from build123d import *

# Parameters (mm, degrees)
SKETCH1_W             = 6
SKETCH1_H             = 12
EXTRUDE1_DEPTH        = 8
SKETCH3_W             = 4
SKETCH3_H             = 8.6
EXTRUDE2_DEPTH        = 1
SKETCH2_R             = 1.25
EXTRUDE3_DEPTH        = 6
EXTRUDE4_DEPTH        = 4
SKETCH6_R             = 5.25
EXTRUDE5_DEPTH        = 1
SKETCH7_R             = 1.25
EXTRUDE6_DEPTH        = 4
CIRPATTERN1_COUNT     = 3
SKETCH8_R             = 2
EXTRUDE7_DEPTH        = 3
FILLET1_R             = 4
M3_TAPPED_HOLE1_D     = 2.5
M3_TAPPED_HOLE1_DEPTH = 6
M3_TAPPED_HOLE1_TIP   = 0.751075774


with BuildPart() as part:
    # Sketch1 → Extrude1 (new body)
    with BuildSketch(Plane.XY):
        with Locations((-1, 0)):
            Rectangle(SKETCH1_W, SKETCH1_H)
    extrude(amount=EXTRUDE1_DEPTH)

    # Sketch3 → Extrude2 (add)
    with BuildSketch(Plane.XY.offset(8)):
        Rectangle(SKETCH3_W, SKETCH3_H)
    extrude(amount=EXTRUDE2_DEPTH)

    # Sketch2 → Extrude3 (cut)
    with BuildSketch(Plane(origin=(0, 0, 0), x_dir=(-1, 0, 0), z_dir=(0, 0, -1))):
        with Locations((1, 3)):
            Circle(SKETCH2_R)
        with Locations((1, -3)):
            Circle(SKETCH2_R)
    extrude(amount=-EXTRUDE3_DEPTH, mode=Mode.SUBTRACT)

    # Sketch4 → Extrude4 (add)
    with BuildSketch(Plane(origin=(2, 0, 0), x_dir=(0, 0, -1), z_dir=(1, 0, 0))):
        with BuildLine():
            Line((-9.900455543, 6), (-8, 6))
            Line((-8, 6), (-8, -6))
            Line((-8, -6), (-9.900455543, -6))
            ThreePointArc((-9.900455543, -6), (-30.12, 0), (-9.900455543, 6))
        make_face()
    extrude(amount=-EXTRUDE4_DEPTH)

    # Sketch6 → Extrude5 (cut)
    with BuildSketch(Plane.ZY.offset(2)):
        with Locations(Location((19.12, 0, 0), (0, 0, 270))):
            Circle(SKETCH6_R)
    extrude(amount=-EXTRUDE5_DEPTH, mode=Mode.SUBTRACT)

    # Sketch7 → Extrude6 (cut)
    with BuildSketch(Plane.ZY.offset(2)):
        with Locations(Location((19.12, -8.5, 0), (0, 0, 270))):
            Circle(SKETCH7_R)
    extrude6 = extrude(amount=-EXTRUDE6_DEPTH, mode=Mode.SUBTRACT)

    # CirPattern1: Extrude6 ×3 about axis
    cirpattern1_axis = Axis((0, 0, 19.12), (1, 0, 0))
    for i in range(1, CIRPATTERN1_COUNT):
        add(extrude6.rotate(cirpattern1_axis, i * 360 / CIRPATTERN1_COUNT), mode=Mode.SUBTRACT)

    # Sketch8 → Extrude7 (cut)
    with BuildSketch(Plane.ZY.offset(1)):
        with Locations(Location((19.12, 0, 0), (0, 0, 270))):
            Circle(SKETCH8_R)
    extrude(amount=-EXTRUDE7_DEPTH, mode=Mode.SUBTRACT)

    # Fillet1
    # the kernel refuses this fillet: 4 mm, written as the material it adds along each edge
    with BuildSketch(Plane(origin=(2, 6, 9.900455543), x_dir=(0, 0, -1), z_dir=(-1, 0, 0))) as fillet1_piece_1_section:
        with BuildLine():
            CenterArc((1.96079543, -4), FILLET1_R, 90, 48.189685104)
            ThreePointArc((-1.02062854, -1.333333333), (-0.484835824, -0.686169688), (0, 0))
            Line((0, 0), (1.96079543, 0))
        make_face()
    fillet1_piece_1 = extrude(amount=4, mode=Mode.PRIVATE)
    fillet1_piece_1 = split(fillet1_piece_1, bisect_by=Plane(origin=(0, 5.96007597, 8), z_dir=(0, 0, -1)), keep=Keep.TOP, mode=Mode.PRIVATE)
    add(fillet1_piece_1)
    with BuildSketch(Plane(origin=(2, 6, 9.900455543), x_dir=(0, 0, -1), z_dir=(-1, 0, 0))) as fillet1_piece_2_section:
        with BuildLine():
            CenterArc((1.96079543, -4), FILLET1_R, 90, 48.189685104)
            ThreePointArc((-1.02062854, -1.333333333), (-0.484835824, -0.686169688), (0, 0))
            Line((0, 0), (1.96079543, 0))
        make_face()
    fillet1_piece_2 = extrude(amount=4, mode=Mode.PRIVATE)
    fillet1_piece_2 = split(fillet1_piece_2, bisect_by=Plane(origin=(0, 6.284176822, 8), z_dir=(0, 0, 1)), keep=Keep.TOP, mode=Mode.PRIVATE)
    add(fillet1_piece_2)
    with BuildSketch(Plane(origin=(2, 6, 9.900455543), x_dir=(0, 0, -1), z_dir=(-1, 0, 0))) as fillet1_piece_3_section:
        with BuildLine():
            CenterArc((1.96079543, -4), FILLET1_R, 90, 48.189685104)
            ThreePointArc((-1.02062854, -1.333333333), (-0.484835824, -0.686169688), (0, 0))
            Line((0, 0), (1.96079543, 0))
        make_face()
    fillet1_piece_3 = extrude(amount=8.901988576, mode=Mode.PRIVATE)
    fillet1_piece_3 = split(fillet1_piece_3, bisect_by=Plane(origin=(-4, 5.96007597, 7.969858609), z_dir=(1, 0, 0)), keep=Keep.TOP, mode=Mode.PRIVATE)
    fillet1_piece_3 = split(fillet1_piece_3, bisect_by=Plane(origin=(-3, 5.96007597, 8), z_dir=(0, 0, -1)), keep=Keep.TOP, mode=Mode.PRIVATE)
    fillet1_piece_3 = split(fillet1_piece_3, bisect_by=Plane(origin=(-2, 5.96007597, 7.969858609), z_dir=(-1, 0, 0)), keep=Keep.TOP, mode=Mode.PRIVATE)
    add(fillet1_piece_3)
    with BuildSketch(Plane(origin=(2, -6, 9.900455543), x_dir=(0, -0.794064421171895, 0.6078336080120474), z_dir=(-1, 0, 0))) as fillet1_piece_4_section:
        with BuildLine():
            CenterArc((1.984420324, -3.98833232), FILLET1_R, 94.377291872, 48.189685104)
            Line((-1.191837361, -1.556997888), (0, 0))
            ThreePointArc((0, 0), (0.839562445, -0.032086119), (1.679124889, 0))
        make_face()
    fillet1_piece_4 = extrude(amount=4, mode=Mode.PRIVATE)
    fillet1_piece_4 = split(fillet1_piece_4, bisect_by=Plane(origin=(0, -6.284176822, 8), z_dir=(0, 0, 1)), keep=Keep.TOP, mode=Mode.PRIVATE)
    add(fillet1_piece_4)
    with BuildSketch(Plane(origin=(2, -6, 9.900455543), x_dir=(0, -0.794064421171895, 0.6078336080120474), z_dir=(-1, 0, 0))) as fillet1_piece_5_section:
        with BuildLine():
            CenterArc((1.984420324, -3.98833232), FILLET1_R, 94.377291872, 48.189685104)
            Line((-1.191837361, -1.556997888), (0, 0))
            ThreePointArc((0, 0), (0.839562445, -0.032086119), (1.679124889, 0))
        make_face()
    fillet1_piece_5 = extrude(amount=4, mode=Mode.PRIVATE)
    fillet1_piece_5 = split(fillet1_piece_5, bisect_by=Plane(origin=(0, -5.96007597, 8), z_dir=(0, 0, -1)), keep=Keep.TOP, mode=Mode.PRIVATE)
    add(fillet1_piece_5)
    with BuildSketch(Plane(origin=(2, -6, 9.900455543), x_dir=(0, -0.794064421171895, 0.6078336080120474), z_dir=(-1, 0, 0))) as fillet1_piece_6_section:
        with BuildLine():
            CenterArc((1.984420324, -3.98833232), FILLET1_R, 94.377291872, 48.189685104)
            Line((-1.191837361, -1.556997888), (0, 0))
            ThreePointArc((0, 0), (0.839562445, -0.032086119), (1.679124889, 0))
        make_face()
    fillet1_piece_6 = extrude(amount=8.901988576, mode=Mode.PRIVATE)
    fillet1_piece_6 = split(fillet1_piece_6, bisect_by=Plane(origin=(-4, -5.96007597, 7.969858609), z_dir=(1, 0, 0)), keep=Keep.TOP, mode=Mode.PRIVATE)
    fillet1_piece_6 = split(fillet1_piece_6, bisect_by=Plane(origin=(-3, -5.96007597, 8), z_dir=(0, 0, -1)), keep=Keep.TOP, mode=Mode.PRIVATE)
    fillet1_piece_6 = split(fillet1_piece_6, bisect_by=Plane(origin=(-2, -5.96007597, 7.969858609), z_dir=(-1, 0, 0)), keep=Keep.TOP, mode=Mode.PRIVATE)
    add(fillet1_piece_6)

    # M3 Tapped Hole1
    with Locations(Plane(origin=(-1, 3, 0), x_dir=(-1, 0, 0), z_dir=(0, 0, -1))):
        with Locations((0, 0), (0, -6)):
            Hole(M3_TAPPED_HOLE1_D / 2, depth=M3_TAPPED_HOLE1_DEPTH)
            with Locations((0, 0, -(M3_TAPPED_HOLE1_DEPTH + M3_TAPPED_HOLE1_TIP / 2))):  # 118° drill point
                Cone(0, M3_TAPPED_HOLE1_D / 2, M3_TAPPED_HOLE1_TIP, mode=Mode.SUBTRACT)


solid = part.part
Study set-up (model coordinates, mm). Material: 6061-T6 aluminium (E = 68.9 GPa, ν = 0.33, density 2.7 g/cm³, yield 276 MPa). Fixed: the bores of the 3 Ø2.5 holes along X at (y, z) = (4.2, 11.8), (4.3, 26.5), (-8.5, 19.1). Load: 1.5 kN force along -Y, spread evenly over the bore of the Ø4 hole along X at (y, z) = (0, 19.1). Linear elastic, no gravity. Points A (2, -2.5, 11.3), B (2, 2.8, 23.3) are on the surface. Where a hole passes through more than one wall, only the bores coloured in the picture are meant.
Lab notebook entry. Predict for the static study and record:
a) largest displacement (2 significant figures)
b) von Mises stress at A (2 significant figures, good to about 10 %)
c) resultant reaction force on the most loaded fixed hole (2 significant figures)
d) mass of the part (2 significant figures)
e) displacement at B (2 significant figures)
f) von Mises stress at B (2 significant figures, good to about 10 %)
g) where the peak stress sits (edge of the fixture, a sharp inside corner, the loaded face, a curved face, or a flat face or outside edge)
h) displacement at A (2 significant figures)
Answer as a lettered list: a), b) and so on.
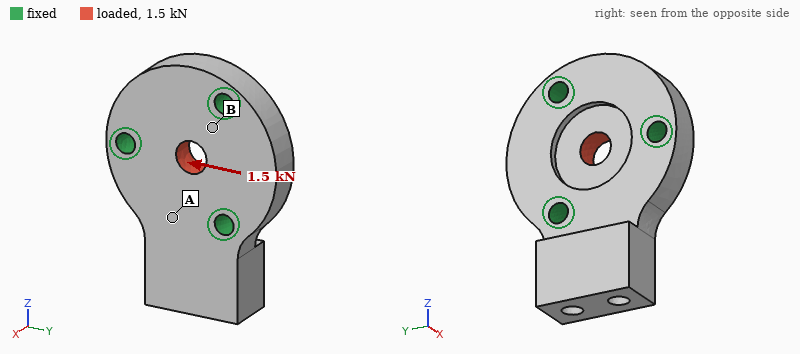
a) 4.4 µm
b) 7.9 MPa
c) 530 N
d) 5.1 g
e) 1.6 µm
f) 22 MPa
g) the loaded face
h) 1.0 µm
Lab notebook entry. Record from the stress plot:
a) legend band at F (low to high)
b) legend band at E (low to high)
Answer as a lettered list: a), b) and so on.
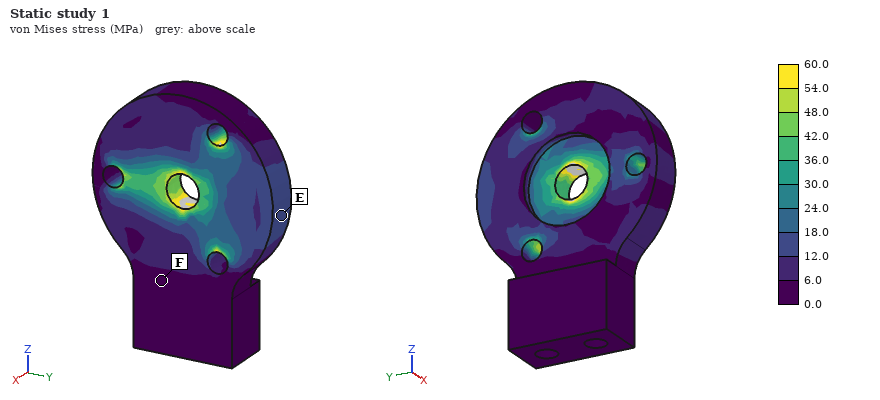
a) 0.0 to 6.0 MPa
b) 12.0 to 18.0 MPa
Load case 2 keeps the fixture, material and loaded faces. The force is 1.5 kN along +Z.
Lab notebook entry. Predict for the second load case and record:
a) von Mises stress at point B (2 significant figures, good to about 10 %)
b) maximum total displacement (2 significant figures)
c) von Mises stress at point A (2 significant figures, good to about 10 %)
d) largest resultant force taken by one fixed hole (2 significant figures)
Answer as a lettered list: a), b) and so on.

a) 34 MPa
b) 4.1 µm
c) 13 MPa
d) 520 N
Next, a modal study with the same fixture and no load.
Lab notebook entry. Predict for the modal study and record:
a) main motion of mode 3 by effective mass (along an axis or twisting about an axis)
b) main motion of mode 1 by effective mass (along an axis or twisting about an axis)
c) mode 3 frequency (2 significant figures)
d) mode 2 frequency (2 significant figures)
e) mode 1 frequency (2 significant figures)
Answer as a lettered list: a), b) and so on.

a) along Y
b) along X
c) 39 kHz
d) 34 kHz
e) 16 kHz
